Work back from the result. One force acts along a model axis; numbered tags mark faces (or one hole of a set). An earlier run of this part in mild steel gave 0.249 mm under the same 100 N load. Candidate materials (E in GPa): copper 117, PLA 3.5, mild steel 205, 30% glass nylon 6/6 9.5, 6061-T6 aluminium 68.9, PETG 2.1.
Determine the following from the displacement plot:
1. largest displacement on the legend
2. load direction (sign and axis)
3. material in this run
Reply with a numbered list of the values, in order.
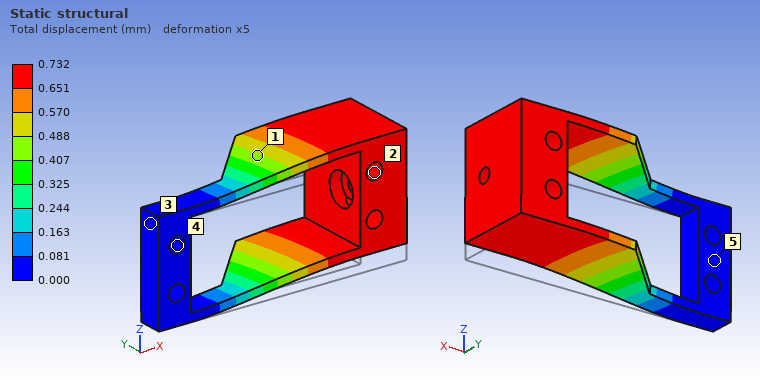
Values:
1. 0.732 mm
2. +Z
3. 6061-T6 aluminium
